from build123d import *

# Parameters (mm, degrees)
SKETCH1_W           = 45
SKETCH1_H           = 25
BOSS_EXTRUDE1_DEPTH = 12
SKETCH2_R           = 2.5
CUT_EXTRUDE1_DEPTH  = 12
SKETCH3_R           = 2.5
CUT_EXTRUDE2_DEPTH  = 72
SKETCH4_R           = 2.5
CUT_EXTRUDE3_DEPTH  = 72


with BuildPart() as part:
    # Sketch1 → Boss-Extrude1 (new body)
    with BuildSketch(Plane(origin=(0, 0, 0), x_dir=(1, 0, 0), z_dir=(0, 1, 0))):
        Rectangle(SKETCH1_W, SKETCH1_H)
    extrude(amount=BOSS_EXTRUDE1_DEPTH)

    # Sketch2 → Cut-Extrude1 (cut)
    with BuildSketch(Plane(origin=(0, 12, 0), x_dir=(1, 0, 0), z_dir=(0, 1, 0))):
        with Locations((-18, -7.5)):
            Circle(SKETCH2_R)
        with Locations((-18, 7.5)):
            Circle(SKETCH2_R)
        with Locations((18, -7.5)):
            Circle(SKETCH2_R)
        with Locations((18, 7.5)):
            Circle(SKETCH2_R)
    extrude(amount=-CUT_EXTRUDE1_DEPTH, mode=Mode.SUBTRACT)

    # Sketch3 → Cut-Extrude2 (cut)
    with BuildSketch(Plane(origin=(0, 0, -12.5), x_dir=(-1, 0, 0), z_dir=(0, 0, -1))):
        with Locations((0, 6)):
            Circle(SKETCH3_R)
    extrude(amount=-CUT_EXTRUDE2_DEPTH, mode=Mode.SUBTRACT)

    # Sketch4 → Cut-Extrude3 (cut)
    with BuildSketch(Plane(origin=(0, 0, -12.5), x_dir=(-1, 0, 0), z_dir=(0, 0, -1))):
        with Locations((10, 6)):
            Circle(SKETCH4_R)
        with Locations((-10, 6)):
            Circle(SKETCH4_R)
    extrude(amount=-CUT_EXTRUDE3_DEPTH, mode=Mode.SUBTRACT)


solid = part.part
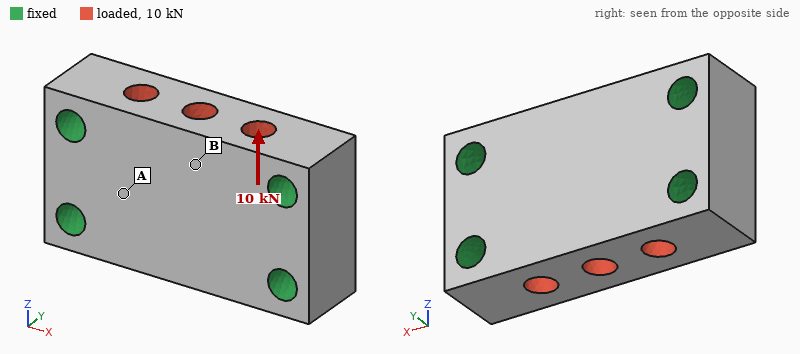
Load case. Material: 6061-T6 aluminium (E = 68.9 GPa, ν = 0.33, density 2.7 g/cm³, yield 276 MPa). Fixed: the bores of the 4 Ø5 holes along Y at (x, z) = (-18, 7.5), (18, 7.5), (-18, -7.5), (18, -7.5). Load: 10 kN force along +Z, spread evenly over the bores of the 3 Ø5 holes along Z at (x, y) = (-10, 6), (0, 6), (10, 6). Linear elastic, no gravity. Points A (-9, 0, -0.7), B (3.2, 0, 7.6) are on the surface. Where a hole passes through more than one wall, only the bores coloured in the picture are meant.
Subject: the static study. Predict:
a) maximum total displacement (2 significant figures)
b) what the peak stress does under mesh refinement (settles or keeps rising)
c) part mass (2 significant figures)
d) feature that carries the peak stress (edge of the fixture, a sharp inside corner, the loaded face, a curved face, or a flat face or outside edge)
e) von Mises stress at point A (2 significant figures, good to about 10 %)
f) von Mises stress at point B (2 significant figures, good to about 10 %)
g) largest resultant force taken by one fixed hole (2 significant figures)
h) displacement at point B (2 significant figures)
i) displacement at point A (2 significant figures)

11 µm
keeps rising
30 g
edge of the fixture
37 MPa
11 MPa
3.0 kN
9.7 µm
6.6 µm
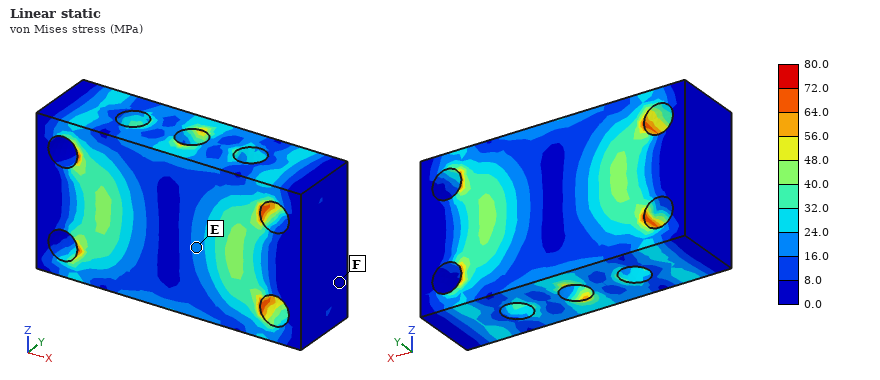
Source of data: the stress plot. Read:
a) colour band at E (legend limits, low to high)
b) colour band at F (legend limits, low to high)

16.0 to 24.0 MPa
0.0 to 8.0 MPa
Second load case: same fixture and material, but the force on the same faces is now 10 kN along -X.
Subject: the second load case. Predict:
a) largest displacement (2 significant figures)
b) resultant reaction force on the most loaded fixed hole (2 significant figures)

4.0 µm
2.5 kN
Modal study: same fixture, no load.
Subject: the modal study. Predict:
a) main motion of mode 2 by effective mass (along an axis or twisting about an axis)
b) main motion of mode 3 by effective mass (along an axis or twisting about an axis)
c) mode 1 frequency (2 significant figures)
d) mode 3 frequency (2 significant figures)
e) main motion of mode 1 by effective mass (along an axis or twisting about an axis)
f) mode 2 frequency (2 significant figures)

twisting about X
along Z
29 kHz
38 kHz
along Y
36 kHz
